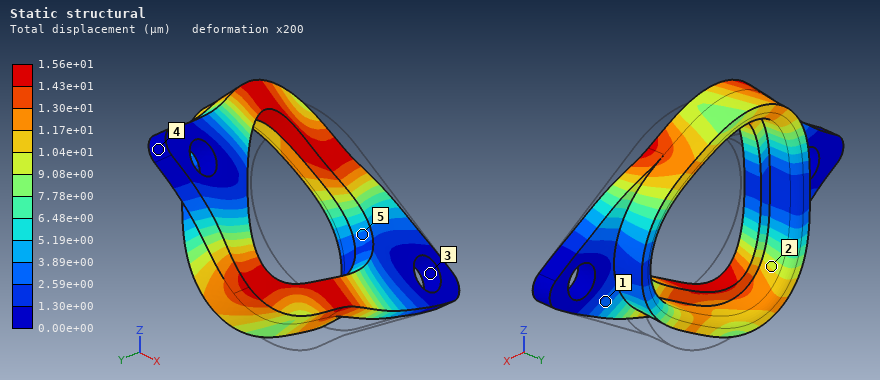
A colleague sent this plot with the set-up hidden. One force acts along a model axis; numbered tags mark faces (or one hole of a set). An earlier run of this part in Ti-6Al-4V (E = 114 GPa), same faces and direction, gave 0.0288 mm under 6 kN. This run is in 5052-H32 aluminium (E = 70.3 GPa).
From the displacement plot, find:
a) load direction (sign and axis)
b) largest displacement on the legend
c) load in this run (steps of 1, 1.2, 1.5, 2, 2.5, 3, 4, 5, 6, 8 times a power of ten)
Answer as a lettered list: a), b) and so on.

a) -X
b) 1.56e+01 µm
c) 2 kN
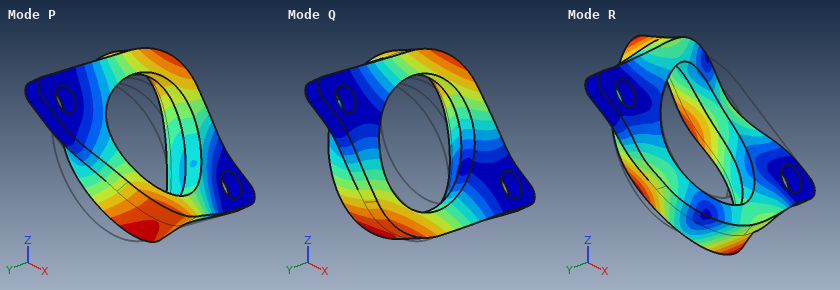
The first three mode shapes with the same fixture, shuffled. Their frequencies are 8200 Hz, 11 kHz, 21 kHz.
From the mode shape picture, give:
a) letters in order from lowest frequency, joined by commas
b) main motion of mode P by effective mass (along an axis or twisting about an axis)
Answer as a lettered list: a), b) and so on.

a) Q, P, R
b) along Y
